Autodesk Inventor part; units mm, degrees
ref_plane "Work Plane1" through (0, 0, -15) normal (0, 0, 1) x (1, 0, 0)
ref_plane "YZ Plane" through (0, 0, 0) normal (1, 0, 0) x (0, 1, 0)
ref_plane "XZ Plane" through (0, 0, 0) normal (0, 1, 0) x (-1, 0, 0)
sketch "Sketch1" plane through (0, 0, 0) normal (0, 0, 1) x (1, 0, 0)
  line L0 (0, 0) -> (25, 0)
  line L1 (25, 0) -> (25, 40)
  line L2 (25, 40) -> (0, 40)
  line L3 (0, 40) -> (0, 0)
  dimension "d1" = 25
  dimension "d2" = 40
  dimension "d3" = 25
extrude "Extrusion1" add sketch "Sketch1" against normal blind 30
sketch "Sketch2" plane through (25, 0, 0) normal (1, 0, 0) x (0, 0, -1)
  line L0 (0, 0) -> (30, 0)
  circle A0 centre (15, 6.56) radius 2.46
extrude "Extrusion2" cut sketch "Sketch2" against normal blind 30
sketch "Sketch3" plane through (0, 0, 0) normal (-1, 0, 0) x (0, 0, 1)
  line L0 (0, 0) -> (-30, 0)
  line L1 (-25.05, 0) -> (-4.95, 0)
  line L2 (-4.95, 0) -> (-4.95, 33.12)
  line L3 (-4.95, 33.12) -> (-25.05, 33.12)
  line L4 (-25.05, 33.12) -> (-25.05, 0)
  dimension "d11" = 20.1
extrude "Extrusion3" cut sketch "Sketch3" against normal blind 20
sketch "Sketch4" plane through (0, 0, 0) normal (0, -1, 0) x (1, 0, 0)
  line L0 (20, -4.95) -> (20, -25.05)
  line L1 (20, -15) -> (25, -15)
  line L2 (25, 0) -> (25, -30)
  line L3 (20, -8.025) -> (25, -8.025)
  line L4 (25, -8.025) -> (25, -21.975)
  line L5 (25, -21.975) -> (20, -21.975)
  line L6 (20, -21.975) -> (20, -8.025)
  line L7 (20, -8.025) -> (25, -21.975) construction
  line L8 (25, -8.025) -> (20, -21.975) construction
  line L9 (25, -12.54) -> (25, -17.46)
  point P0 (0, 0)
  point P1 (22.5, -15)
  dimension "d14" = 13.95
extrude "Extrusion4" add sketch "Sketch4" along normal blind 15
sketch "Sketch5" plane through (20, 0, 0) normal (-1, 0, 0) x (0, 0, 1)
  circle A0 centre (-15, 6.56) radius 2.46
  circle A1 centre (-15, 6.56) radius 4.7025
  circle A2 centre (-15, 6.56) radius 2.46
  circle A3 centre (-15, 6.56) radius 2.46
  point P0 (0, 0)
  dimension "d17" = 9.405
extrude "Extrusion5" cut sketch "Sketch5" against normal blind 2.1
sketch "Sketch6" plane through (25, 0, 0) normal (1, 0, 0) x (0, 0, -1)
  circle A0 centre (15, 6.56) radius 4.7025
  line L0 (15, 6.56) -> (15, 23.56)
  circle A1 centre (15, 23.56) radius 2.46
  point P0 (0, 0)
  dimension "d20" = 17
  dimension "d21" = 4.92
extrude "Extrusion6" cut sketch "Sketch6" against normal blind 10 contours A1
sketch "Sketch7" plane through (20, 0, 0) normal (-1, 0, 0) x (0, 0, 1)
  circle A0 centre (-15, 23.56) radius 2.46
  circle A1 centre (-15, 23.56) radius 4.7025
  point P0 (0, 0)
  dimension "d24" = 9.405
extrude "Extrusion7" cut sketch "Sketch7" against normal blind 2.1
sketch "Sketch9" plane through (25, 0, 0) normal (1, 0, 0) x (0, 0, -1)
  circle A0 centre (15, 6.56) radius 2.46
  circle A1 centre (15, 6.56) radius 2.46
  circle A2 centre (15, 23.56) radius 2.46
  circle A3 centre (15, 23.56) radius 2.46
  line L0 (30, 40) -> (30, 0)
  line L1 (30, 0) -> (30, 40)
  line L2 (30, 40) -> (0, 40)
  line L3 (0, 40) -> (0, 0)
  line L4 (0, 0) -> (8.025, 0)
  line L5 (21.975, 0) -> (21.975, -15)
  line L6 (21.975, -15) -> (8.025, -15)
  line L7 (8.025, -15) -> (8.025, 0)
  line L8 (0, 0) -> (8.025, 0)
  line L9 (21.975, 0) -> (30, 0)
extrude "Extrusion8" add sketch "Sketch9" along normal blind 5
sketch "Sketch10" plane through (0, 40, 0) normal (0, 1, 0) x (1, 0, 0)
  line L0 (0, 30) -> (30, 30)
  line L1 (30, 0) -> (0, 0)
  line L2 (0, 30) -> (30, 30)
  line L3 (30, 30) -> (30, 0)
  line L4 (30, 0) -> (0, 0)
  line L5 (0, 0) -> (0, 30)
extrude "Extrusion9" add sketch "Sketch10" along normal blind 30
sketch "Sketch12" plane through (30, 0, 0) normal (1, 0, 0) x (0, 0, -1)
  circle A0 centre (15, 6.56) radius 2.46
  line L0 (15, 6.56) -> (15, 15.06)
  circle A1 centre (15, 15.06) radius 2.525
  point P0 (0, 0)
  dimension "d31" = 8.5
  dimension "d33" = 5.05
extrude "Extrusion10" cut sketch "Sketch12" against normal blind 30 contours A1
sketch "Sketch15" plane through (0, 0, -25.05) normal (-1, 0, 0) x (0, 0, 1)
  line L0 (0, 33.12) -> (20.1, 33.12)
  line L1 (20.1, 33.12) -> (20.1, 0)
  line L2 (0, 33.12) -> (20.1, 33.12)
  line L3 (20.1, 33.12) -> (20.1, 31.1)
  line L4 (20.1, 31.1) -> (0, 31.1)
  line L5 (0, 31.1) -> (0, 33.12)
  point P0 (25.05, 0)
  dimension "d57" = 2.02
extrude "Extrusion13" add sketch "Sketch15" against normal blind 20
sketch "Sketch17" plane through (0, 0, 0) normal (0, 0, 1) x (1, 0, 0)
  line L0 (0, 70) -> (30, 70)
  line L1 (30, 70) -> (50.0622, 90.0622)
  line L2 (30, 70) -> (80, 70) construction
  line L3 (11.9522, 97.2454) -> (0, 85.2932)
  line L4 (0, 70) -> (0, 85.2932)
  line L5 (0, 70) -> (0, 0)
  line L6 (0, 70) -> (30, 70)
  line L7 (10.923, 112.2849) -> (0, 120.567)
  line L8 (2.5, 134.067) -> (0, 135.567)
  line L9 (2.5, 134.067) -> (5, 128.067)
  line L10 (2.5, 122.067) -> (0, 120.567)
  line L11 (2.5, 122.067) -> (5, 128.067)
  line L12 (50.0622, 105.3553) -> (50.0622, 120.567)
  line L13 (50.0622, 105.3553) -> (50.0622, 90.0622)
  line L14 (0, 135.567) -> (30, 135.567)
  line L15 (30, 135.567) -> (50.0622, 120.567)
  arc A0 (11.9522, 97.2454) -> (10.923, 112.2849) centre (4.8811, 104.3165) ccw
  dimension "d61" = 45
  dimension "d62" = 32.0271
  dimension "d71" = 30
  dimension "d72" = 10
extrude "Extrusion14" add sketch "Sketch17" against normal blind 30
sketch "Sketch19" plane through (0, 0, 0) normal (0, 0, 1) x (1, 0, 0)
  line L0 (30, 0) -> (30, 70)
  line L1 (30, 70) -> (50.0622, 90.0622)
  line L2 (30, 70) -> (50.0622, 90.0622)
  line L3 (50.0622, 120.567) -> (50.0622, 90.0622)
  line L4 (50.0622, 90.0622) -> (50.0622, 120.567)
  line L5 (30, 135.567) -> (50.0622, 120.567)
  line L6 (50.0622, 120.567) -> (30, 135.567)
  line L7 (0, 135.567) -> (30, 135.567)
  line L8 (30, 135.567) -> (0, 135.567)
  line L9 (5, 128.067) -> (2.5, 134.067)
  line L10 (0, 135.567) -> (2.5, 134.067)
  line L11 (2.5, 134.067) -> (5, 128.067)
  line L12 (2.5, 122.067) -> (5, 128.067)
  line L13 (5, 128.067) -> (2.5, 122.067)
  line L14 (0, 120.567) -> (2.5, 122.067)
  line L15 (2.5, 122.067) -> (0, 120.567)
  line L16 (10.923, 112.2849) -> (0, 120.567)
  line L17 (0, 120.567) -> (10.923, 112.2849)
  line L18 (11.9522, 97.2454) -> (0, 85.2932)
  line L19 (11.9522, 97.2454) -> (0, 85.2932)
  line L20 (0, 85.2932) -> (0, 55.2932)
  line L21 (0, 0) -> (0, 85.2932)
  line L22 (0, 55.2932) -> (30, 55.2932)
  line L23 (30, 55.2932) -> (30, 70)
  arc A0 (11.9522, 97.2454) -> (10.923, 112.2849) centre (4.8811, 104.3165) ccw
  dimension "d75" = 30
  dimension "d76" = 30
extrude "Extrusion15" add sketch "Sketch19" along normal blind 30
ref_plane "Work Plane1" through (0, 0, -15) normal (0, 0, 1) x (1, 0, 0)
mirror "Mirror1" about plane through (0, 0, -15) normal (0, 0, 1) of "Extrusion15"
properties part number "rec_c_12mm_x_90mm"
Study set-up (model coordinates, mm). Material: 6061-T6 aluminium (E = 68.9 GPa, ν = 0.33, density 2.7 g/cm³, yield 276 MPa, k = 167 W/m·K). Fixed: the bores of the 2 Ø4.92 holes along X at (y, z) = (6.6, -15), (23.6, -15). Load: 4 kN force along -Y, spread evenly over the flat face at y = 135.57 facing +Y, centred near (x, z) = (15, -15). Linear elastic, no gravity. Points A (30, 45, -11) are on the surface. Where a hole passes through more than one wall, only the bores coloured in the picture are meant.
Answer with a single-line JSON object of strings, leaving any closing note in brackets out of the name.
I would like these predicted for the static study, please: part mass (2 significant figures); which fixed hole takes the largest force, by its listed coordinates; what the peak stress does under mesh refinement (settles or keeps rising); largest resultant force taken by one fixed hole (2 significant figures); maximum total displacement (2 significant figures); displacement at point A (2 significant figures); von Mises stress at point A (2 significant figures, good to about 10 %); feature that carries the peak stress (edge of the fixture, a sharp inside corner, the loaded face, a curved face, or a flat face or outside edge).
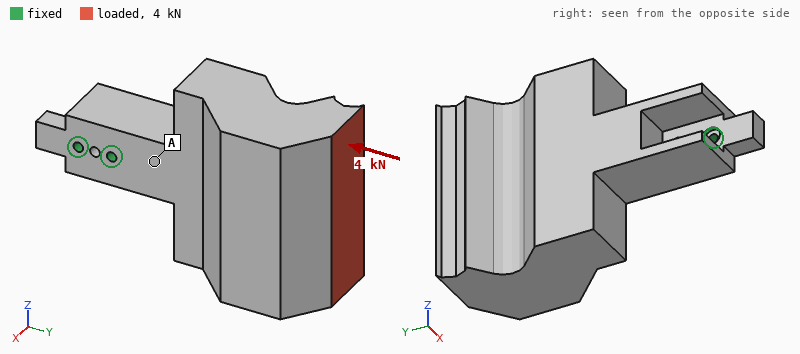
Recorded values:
{"part mass": "830 g", "which fixed hole takes the largest force, by its listed coordinates": "(23.6, -15)", "what the peak stress does under mesh refinement": "keeps rising", "largest resultant force taken by one fixed hole": "3.0 kN", "maximum total displacement": "0.11 mm", "displacement at point A": "0.020 mm", "von Mises stress at point A": "5.5 MPa", "feature that carries the peak stress": "edge of the fixture"}
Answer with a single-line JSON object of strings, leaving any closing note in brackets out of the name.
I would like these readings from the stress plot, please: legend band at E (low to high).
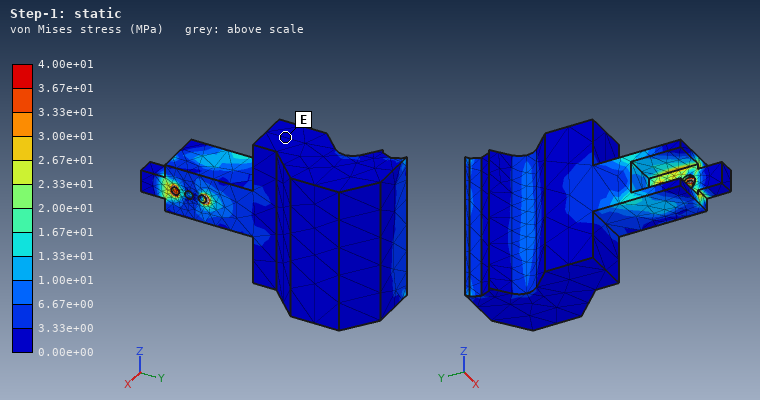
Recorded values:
{"legend band at E": "0.00e+00 to 3.33e+00 MPa"}
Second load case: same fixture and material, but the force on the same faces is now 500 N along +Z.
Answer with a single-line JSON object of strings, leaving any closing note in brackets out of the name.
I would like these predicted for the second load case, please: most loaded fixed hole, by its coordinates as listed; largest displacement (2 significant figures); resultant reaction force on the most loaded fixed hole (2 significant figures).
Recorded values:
{"most loaded fixed hole, by its coordinates as listed": "(23.6, -15)", "largest displacement": "0.14 mm", "resultant reaction force on the most loaded fixed hole": "2.9 kN"}
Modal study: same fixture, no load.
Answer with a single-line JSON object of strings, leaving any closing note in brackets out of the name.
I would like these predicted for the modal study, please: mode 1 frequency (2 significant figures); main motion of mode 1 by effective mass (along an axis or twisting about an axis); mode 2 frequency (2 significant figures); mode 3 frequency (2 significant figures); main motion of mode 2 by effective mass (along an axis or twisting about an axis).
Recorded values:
{"mode 1 frequency": "460 Hz", "main motion of mode 1 by effective mass": "along X", "mode 2 frequency": "510 Hz", "mode 3 frequency": "860 Hz", "main motion of mode 2 by effective mass": "along Z"}
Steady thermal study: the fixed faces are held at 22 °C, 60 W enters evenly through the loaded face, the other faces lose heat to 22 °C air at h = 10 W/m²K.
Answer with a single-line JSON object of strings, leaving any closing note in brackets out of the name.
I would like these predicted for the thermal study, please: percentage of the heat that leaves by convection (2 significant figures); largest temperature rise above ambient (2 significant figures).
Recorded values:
{"percentage of the heat that leaves by convection": "13 %", "largest temperature rise above ambient": "35 K"}
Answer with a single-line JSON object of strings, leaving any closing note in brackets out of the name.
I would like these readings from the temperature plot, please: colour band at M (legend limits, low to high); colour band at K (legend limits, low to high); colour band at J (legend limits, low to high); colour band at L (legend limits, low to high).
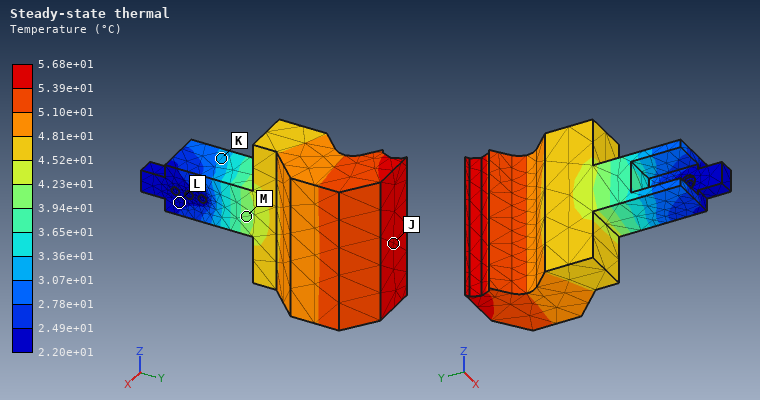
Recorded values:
{"colour band at M": "3.94e+01 to 4.23e+01 °C", "colour band at K": "3.07e+01 to 3.36e+01 °C", "colour band at J": "5.39e+01 to 5.68e+01 °C", "colour band at L": "2.20e+01 to 2.49e+01 °C"}
